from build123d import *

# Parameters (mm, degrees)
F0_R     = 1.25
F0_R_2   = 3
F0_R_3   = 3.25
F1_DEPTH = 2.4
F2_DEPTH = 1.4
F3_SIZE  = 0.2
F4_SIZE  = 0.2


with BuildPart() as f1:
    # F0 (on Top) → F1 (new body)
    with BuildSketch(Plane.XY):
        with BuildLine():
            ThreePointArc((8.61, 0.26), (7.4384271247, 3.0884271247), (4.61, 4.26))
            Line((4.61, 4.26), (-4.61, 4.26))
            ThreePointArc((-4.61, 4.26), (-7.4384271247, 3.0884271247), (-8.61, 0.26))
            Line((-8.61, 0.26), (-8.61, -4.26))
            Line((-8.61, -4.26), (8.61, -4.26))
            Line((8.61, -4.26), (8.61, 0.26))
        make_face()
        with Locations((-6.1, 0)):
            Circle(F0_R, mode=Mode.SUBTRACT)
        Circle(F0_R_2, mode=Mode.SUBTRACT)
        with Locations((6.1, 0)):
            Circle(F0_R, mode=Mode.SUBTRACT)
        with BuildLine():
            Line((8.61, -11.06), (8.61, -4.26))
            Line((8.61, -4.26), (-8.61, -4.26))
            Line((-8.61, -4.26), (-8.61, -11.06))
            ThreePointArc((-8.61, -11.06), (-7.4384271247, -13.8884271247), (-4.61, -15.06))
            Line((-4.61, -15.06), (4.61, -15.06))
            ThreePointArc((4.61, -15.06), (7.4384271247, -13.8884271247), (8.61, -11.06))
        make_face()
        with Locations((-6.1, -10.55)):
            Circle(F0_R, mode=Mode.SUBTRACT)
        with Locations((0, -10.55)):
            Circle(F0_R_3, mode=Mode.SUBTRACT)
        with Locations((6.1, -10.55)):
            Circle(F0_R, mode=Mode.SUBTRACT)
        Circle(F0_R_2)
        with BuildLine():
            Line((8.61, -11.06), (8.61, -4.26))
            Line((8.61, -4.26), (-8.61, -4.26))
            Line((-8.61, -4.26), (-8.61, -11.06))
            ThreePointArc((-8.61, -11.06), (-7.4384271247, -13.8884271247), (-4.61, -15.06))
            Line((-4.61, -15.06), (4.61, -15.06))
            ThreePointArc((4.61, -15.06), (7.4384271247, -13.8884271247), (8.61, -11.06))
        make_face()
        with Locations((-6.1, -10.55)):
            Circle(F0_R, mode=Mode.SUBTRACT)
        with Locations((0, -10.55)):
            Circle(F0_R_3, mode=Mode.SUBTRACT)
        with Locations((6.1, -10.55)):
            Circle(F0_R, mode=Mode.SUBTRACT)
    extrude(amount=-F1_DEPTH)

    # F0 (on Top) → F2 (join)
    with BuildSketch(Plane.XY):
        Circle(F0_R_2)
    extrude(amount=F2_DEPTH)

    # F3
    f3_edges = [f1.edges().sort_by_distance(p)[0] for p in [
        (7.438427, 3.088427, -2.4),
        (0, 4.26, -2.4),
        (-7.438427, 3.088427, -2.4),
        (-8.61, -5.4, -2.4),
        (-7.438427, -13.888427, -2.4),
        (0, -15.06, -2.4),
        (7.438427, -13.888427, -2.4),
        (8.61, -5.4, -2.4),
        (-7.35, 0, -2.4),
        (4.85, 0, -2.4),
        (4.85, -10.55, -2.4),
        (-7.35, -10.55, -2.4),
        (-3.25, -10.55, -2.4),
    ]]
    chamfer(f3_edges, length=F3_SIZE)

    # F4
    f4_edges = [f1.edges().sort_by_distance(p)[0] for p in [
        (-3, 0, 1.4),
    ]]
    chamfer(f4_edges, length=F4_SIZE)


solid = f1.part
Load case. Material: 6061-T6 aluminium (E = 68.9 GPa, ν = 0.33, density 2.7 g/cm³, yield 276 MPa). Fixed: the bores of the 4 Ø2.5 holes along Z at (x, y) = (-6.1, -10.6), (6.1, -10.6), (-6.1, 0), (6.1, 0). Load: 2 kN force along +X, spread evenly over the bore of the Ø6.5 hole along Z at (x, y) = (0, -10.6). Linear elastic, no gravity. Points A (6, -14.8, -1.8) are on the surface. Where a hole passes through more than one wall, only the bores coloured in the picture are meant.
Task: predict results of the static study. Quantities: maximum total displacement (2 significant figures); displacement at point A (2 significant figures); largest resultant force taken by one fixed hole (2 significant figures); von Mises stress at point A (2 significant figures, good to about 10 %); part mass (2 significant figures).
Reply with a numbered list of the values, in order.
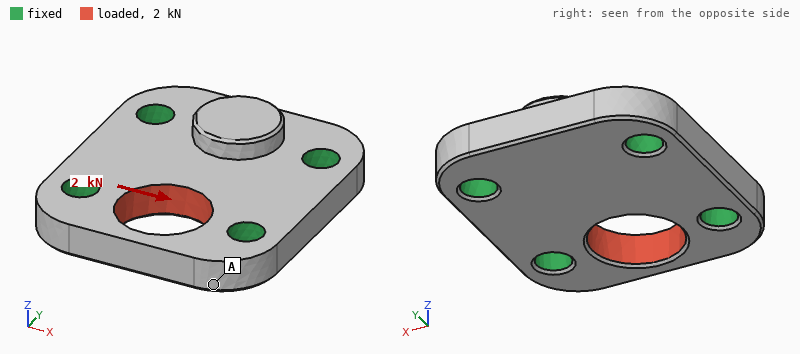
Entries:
1. 8.7 µm
2. 5.3 µm
3. 870 N
4. 17 MPa
5. 1.8 g
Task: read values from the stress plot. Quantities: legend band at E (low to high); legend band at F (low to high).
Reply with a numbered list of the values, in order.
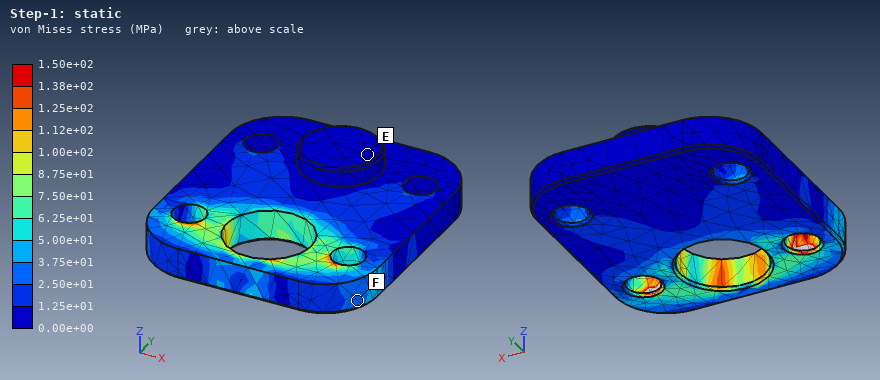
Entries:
1. 0.00e+00 to 1.25e+01 MPa
2. 2.50e+01 to 3.75e+01 MPa
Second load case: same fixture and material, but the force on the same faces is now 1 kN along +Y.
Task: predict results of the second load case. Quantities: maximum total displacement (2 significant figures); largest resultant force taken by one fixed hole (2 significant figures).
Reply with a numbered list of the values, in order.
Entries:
1. 9.0 µm
2. 370 N
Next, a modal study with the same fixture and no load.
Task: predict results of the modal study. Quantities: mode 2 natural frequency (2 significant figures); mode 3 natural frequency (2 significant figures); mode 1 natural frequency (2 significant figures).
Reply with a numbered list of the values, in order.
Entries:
1. 69 kHz
2. 70 kHz
3. 67 kHz
